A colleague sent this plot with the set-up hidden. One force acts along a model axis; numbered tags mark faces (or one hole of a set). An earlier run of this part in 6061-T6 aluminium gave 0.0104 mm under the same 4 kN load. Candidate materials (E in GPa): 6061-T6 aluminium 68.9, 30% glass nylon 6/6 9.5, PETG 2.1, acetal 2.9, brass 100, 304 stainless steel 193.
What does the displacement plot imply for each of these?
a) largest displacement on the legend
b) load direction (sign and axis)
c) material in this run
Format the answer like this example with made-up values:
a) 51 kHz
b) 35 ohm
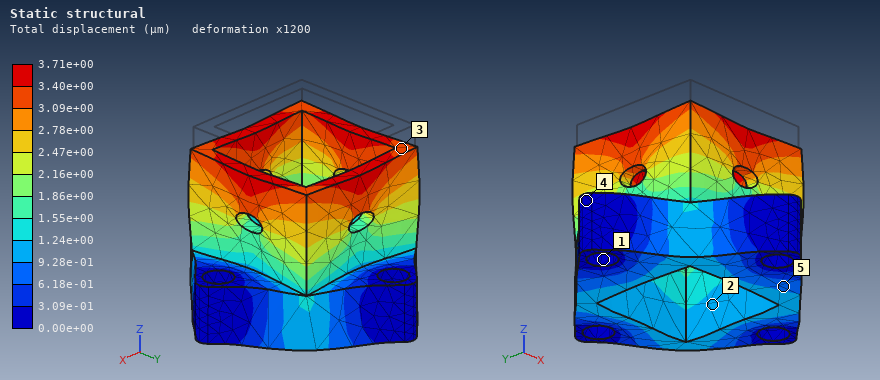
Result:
a) 3.71e+00 µm
b) -Z
c) 304 stainless steel
